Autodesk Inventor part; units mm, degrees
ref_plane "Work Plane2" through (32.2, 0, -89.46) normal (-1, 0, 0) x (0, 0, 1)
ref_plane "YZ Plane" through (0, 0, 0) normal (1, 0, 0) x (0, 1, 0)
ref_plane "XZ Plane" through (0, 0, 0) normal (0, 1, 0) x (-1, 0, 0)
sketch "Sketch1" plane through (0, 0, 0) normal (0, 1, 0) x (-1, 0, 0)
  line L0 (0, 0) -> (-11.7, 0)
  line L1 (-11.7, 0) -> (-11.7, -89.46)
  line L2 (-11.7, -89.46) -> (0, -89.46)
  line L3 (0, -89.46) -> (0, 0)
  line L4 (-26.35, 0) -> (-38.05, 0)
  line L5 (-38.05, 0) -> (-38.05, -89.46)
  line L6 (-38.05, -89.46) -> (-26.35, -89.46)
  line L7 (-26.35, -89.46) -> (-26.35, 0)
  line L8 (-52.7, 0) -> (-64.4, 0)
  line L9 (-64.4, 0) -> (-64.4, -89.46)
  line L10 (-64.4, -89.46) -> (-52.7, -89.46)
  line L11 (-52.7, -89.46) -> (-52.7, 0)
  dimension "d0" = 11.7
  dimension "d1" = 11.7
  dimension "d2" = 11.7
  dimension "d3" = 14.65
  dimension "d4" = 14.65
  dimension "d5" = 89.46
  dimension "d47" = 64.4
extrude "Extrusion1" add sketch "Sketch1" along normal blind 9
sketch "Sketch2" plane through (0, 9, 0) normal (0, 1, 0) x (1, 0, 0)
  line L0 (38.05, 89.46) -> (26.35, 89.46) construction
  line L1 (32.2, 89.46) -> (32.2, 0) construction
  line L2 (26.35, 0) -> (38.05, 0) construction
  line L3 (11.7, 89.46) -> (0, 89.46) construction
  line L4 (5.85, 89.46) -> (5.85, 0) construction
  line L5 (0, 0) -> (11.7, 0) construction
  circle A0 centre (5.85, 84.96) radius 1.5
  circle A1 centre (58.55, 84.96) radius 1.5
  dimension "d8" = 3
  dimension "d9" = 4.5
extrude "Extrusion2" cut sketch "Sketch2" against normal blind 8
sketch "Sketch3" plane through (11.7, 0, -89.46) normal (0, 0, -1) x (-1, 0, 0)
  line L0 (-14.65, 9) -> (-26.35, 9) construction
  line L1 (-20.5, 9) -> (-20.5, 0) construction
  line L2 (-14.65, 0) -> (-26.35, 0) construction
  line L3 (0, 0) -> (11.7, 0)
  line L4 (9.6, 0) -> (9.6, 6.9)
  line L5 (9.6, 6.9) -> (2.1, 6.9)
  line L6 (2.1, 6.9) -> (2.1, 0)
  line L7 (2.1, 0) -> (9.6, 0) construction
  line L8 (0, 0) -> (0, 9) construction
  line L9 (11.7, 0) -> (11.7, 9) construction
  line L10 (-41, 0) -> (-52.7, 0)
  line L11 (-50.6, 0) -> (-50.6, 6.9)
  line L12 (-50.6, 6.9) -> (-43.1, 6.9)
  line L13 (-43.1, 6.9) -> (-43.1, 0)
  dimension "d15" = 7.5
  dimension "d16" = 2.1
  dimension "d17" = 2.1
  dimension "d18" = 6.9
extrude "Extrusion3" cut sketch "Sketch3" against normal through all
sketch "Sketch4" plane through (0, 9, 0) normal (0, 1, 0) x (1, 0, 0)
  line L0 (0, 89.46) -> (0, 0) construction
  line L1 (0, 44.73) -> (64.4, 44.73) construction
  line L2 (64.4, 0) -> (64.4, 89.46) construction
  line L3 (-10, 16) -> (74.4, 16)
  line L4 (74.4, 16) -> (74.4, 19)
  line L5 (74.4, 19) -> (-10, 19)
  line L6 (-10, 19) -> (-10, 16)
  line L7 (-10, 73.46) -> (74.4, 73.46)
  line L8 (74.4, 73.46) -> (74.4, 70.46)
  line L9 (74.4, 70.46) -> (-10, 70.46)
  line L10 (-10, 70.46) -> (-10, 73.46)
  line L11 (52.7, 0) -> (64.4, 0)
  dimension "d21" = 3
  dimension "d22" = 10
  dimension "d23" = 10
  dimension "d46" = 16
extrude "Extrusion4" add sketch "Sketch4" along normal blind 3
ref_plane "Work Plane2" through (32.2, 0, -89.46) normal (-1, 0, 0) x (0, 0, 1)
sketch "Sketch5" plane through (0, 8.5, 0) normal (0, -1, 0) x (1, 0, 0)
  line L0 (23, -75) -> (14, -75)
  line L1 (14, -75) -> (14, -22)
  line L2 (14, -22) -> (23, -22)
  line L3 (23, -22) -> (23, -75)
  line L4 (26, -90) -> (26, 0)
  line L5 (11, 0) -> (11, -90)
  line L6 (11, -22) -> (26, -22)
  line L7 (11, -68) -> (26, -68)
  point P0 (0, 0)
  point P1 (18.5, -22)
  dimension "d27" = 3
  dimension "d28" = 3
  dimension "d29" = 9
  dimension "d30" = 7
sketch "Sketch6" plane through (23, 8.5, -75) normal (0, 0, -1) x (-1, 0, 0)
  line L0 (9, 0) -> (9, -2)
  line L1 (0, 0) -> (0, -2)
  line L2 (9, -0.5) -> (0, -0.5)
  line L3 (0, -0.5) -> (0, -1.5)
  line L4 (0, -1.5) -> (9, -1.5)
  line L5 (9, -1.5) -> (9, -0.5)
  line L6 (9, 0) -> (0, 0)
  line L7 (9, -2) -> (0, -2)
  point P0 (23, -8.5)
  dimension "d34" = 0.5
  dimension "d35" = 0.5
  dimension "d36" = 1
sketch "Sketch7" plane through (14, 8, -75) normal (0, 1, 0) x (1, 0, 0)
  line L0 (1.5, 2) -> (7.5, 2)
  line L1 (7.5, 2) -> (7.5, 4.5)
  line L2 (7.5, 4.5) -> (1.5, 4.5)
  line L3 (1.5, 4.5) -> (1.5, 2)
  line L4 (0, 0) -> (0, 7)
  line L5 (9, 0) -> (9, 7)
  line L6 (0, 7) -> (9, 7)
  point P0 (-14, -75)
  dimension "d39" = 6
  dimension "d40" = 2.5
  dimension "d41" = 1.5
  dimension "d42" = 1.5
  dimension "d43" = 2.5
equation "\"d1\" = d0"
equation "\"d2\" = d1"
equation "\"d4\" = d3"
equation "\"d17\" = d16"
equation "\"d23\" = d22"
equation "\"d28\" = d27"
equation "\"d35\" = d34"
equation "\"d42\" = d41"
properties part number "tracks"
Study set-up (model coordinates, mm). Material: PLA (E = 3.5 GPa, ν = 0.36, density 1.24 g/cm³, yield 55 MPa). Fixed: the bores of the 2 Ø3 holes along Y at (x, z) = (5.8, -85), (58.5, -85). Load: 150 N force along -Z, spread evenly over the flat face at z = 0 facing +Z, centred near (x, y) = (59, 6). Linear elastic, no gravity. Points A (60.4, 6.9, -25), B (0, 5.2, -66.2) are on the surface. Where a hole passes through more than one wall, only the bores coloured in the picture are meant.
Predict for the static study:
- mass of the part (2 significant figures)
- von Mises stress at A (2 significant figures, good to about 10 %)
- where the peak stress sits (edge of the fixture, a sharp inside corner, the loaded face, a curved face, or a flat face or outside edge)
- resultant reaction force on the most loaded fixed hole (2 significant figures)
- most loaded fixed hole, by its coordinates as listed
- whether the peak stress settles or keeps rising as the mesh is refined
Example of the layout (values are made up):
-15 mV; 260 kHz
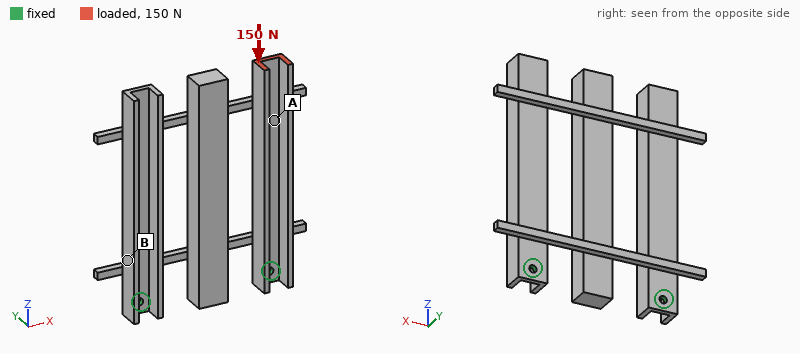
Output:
25 g; 3.0 MPa; edge of the fixture; 150 N; (58.5, -85); keeps rising
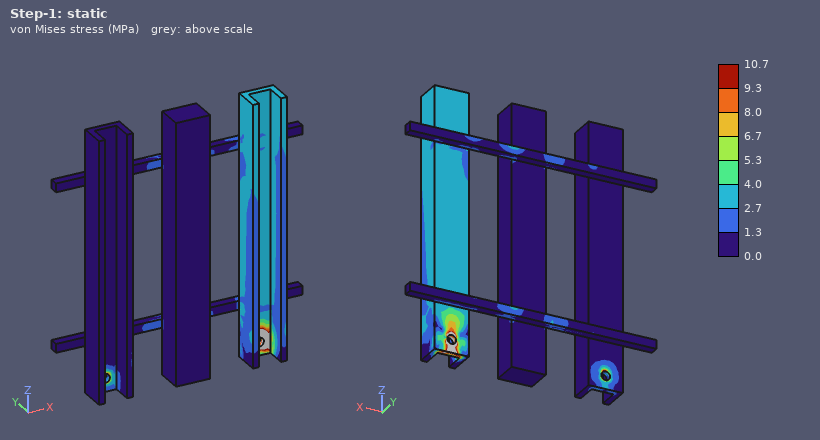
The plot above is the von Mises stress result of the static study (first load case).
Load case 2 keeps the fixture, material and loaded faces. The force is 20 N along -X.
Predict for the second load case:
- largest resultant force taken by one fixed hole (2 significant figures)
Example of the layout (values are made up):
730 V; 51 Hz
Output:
21 N
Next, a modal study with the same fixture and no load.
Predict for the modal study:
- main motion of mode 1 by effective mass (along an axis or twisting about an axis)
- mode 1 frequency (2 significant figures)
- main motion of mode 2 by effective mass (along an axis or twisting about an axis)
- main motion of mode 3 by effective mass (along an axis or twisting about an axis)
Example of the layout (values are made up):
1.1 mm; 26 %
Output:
along Y; 130 Hz; along X; along X
